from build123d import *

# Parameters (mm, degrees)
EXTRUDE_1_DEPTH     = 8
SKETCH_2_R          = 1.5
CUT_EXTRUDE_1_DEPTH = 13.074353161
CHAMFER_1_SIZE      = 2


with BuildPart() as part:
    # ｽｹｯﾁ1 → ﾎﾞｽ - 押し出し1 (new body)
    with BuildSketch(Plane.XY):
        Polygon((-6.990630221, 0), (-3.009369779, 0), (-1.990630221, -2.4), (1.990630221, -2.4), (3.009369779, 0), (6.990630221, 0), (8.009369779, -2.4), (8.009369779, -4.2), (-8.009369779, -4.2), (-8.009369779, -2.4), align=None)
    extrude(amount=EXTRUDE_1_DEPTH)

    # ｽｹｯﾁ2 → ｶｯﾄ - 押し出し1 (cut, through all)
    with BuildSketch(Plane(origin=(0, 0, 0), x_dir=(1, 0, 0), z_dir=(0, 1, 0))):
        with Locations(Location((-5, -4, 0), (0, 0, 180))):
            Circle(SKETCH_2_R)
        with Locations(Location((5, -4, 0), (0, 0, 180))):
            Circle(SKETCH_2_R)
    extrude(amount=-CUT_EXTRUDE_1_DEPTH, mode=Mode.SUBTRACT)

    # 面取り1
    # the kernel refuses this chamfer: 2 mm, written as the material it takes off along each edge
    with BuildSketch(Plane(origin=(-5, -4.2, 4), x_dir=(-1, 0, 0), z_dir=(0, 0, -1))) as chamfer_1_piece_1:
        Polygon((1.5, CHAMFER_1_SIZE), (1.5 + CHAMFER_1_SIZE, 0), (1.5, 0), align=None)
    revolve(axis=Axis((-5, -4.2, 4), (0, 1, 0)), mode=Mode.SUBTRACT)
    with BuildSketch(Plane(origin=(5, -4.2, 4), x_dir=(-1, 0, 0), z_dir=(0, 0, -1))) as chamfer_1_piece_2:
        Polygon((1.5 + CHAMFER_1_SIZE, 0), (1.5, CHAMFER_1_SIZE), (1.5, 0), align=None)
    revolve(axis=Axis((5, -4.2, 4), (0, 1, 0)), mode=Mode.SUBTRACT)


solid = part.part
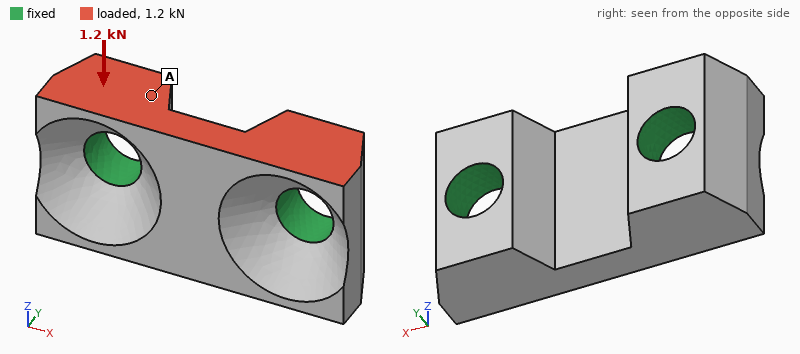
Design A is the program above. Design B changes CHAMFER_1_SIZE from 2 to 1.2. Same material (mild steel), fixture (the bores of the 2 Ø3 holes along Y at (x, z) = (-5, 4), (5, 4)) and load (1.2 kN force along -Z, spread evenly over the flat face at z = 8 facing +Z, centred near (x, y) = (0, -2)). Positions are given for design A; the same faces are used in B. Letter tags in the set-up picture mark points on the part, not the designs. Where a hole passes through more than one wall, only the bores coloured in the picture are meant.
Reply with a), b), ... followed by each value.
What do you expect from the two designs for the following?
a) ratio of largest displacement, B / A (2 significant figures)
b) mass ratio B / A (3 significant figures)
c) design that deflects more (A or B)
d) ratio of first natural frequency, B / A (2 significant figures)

a) 0.44
b) 1.12
c) A
d) 1.3
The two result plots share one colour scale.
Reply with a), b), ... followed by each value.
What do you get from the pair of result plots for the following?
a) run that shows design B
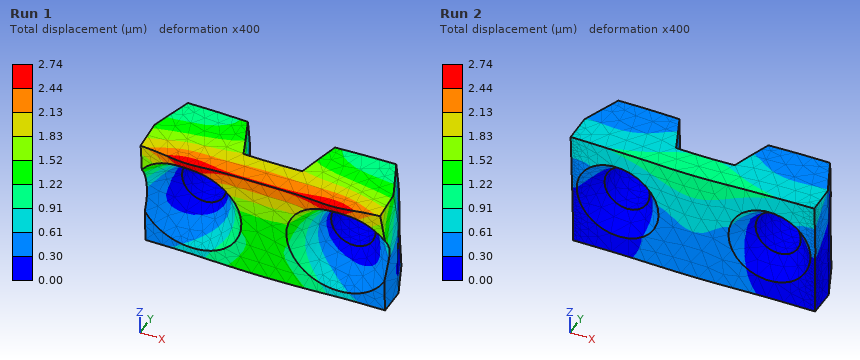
a) Run 2
